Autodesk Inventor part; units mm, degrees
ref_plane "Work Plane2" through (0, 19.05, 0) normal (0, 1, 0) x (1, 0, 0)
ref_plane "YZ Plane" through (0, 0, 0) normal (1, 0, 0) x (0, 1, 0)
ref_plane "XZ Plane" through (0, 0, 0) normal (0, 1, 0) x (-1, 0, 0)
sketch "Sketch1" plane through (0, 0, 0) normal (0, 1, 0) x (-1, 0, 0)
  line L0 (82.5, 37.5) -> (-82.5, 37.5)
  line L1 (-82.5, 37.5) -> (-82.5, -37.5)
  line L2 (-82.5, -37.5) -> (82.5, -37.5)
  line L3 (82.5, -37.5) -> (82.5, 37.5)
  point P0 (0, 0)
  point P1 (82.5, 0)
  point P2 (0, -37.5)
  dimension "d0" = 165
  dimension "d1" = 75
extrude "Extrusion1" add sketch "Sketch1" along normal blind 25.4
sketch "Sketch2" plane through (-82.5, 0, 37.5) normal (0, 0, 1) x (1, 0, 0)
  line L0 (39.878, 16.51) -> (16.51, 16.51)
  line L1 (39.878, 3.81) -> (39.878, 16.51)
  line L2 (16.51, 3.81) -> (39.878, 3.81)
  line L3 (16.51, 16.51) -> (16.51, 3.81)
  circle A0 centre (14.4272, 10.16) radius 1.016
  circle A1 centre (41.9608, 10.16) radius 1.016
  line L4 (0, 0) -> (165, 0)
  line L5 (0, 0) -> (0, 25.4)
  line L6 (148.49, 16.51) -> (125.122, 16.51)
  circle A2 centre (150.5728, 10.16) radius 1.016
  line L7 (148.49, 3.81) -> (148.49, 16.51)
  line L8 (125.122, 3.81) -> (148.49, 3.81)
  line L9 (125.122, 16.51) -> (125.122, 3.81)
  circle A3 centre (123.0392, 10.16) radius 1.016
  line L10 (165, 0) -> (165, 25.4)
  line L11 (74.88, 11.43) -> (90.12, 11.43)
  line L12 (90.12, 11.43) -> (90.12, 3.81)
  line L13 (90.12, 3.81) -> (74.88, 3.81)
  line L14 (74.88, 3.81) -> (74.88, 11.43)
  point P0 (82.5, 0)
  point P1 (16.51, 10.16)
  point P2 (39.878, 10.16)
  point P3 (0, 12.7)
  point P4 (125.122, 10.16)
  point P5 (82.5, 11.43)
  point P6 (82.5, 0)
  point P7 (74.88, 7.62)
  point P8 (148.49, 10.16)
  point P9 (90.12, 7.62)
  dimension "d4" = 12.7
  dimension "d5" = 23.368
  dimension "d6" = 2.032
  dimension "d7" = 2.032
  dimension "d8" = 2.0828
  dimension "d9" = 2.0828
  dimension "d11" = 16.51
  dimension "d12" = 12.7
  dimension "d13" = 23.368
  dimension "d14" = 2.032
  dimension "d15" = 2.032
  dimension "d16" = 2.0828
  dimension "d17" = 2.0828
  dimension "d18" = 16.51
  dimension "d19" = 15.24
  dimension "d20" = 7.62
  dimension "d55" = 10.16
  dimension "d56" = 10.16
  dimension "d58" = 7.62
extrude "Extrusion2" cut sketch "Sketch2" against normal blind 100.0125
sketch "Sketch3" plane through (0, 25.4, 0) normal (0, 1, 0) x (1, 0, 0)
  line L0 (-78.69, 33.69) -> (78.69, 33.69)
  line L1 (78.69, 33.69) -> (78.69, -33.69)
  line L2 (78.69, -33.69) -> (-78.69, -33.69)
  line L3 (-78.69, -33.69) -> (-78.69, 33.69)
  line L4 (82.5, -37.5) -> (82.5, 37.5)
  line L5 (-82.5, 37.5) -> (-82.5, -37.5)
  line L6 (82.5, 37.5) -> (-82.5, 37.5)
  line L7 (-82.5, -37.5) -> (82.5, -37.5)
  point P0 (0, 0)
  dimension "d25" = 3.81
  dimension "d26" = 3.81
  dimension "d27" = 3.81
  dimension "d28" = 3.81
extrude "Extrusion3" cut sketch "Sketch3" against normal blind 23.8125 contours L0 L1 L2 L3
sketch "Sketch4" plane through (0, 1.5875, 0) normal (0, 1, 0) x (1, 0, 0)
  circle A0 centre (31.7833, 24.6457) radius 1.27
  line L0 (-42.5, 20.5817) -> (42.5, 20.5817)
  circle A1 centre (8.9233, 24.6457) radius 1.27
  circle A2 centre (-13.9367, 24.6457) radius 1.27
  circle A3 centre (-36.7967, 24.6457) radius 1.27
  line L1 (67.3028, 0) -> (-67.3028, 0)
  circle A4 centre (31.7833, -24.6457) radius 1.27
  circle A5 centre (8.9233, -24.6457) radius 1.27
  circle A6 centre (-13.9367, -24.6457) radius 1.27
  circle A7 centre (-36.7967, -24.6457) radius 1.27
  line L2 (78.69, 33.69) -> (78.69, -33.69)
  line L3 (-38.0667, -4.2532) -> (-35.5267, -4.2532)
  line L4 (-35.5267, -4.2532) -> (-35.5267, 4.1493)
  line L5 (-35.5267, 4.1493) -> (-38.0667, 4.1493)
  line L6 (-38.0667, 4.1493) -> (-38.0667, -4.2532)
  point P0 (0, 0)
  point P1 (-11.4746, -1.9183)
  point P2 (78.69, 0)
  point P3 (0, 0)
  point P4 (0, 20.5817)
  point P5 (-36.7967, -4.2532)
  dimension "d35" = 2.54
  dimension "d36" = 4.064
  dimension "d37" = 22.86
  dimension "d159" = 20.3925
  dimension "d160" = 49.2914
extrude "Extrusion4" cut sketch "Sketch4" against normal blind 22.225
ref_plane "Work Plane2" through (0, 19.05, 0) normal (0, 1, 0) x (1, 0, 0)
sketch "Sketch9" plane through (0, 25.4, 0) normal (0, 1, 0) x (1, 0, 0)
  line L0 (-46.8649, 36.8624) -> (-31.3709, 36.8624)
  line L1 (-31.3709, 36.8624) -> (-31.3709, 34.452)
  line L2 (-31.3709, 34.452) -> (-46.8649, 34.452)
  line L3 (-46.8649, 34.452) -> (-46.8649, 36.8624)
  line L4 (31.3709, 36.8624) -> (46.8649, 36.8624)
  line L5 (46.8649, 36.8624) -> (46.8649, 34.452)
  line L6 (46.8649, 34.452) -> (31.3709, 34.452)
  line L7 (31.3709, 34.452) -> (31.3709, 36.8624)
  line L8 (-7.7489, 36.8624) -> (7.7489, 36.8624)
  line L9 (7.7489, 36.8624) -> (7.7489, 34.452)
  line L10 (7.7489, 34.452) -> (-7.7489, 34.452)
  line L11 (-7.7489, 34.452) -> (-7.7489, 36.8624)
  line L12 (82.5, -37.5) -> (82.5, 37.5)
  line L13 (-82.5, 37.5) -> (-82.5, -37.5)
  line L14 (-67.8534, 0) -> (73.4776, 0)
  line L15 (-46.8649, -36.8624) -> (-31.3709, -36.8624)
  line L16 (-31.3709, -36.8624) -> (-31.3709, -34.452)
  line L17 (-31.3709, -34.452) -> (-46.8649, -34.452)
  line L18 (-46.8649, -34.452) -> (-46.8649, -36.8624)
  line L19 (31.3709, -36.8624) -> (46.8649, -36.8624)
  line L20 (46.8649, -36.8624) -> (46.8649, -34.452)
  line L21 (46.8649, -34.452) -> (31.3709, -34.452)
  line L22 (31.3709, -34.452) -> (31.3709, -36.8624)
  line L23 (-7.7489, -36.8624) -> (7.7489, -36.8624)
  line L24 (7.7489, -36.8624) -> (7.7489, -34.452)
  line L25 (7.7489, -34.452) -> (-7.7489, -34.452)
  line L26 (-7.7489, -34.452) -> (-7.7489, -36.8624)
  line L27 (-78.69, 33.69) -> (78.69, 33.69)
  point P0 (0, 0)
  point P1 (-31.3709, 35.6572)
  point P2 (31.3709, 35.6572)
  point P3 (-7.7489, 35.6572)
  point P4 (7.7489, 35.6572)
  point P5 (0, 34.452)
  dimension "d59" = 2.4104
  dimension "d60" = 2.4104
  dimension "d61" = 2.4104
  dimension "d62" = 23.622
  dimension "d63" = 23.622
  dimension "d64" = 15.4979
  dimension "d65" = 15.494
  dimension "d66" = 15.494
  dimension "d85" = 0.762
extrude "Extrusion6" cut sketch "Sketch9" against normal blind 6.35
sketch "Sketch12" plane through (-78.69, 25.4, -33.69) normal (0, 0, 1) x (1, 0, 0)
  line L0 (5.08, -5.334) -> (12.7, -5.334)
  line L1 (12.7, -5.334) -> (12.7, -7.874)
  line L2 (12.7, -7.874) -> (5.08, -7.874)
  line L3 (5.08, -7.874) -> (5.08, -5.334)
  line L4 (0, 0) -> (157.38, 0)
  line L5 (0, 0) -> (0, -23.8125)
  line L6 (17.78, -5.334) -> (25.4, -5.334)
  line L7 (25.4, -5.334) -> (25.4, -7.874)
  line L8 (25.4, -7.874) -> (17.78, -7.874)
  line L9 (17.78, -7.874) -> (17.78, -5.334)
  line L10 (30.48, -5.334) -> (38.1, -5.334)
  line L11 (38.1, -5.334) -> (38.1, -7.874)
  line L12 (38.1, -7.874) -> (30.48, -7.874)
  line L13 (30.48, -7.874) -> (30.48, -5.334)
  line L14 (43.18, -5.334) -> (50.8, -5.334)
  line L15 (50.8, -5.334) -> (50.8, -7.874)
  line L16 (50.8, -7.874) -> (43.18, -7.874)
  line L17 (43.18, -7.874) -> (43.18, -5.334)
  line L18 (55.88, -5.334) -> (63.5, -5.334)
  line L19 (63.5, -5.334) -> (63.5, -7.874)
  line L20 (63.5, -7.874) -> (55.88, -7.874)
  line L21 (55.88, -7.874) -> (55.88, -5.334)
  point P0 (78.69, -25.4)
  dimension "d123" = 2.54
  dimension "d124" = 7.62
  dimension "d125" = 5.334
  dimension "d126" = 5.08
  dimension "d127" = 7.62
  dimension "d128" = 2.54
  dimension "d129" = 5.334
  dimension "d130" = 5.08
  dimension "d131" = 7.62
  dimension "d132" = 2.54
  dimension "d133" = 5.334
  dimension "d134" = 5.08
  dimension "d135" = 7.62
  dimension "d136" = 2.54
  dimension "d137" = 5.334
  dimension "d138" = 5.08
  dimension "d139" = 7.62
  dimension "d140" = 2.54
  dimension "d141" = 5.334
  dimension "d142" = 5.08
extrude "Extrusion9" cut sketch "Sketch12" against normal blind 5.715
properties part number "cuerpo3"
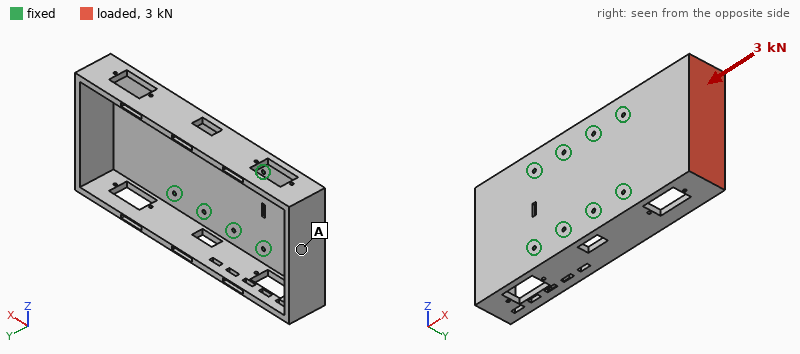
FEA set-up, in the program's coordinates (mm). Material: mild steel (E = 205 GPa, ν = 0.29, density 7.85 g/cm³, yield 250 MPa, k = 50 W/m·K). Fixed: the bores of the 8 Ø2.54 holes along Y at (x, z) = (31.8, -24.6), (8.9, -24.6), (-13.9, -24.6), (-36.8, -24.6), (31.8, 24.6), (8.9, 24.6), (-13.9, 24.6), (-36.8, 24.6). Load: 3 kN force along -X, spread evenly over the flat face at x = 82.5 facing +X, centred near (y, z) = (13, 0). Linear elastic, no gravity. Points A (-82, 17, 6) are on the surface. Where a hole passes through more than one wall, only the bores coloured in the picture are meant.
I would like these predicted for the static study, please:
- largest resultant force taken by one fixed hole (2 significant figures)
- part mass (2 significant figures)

620 N
430 g
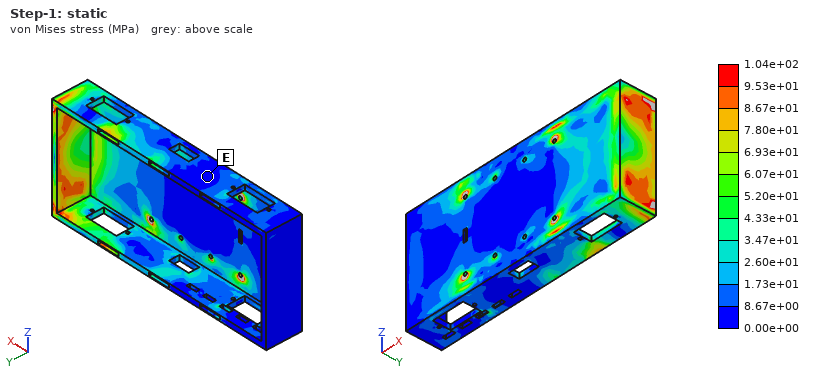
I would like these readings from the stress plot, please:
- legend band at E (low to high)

0.00e+00 to 8.67e+00 MPa
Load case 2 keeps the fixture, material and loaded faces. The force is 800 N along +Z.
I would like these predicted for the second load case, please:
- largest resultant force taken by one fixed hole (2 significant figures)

780 N
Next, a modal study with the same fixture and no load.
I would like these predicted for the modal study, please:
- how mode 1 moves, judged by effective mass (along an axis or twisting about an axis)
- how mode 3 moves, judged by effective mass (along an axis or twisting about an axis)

twisting about Z
along Z
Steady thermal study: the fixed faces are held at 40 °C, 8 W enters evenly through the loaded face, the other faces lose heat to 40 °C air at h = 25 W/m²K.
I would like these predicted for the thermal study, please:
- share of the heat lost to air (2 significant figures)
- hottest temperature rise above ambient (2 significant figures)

68 %
27 K
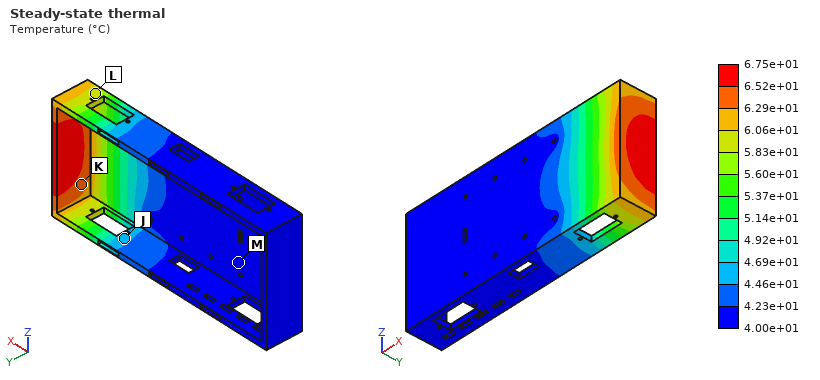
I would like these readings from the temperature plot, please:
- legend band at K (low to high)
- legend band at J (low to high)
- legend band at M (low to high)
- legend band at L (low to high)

6.29e+01 to 6.52e+01 °C
4.46e+01 to 4.69e+01 °C
4.00e+01 to 4.23e+01 °C
5.83e+01 to 6.06e+01 °C
